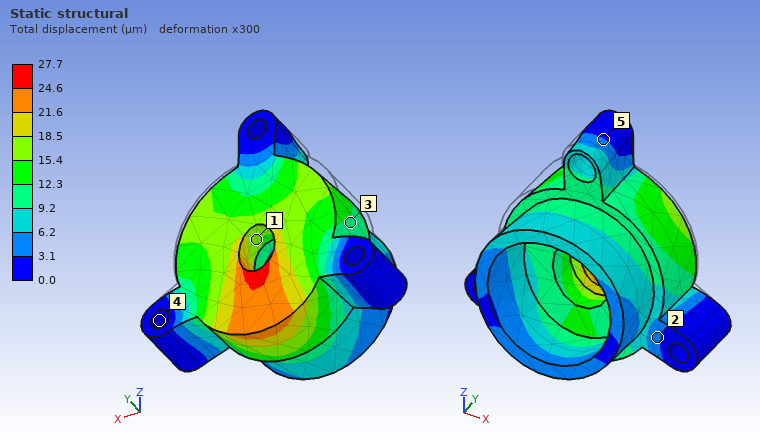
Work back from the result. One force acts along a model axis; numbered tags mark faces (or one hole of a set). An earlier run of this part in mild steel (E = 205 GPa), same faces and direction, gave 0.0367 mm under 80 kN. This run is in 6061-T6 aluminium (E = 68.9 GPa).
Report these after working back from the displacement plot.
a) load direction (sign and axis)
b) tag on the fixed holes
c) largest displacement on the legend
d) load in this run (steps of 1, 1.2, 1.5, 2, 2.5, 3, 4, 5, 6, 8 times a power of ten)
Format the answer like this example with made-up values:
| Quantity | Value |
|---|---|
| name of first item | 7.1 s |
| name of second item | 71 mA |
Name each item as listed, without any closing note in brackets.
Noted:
| Quantity | Value |
|---|---|
| load direction | -Z |
| tag on the fixed holes | 4 |
| largest displacement on the legend | 27.7 µm |
| load in this run | 20 kN |
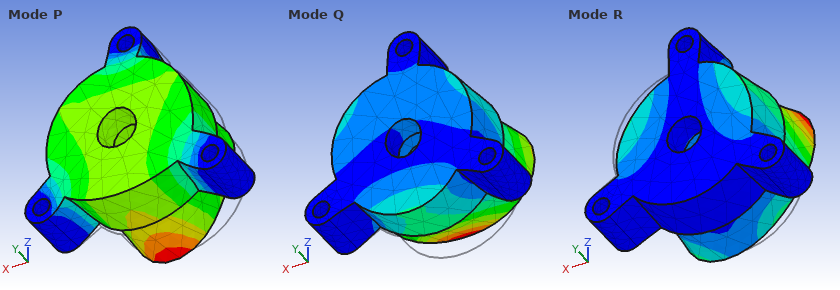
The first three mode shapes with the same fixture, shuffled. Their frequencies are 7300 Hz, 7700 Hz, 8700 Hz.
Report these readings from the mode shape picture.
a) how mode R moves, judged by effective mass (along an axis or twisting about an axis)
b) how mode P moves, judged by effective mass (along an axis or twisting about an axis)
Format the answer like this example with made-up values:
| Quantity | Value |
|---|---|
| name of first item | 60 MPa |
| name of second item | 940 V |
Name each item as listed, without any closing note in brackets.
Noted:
| Quantity | Value |
|---|---|
| how mode R moves, judged by effective mass | along X |
| how mode P moves, judged by effective mass | along Y |
